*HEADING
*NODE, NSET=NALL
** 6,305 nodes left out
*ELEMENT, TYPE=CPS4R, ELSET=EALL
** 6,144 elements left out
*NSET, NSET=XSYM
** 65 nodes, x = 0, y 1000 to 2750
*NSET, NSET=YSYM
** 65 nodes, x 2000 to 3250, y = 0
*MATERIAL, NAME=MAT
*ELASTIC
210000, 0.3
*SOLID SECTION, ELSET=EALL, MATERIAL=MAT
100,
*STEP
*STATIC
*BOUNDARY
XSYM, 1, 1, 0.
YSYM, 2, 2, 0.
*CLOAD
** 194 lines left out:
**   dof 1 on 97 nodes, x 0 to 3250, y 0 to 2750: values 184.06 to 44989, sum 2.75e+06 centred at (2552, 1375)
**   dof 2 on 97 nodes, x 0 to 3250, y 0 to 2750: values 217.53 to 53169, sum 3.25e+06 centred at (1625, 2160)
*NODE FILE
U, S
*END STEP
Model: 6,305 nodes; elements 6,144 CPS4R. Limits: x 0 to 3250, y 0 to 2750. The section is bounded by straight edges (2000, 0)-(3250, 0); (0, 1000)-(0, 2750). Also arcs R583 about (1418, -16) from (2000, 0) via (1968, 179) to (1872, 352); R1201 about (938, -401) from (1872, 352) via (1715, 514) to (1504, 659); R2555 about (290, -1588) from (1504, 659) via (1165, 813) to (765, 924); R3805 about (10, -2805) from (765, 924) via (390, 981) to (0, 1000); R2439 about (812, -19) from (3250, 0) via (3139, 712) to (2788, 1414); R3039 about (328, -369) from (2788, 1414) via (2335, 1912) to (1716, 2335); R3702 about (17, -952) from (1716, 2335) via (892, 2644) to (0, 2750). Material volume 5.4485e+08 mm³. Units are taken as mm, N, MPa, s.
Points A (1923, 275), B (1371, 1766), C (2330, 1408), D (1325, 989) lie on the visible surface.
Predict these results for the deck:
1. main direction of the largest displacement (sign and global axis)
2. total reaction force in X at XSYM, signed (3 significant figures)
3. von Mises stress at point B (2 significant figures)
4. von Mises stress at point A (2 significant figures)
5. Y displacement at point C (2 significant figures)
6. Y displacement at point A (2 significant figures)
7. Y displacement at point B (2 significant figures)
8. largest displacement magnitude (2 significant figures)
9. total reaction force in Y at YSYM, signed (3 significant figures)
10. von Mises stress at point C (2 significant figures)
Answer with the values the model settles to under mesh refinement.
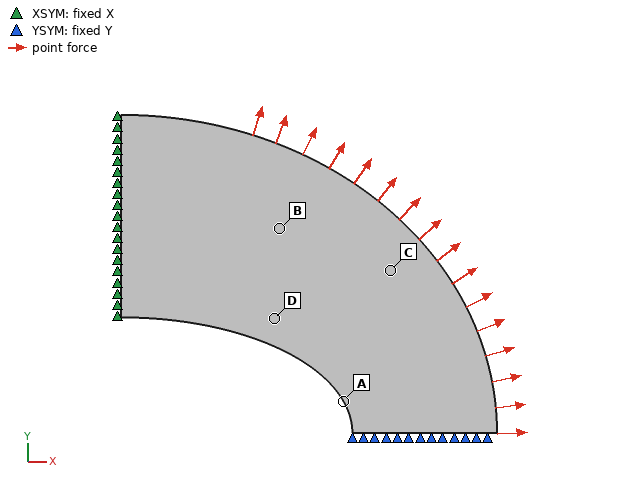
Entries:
+Y
-2.75e+06 N
19 MPa
70 MPa
0.16 mm
0.12 mm
0.40 mm
0.55 mm
-3.25e+06 N
17 MPa
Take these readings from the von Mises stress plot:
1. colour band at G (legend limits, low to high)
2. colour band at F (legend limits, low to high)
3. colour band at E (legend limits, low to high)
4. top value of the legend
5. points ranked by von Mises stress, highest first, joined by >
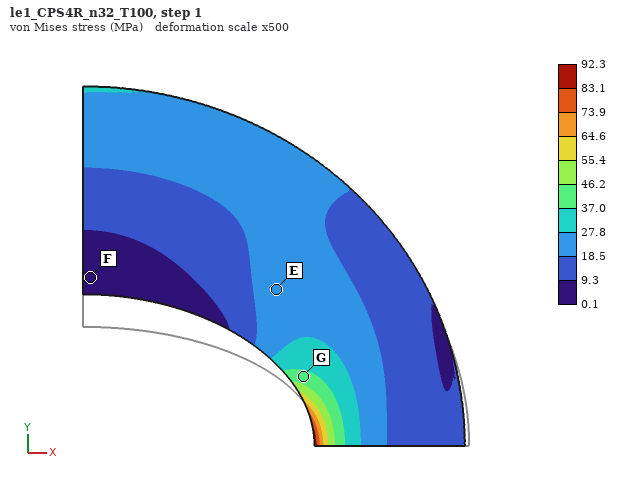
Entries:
37.0 to 46.2 MPa
0.1 to 9.3 MPa
18.5 to 27.8 MPa
92.3 MPa
G > E > F
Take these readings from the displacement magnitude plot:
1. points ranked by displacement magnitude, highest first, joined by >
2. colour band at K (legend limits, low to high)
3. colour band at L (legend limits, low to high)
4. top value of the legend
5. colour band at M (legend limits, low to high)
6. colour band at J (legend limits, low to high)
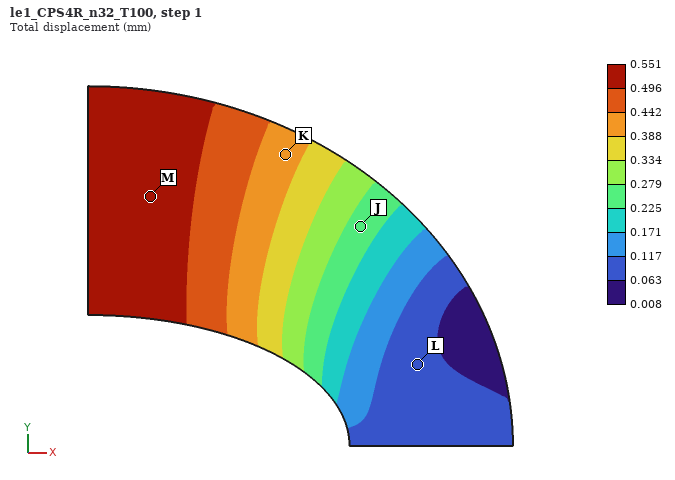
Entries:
M > K > J > L
0.388 to 0.442 mm
0.063 to 0.117 mm
0.551 mm
0.496 to 0.551 mm
0.225 to 0.279 mm
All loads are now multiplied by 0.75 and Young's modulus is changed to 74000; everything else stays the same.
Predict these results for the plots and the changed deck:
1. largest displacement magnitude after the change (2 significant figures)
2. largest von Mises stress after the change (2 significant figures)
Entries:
1.2 mm
69 MPa
